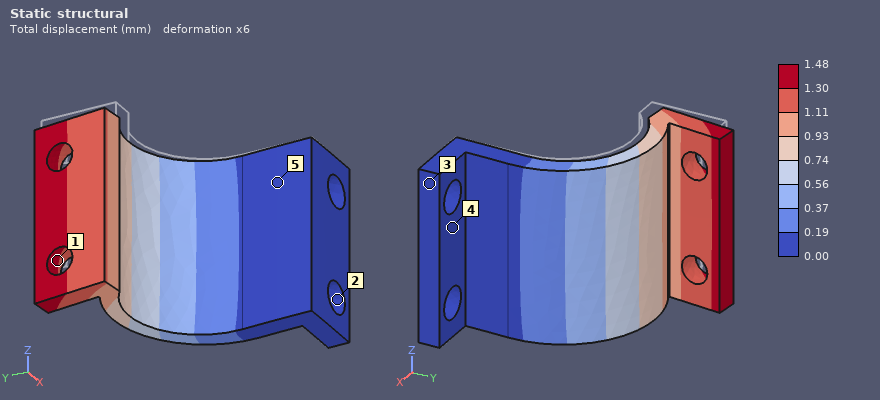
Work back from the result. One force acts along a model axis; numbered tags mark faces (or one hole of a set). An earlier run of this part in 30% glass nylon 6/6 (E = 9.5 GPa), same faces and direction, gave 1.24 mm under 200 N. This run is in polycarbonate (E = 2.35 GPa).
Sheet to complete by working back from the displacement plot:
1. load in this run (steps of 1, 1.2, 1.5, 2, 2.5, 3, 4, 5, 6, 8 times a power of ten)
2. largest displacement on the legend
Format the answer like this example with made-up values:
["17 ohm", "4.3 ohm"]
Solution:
["60 N", "1.48 mm"]
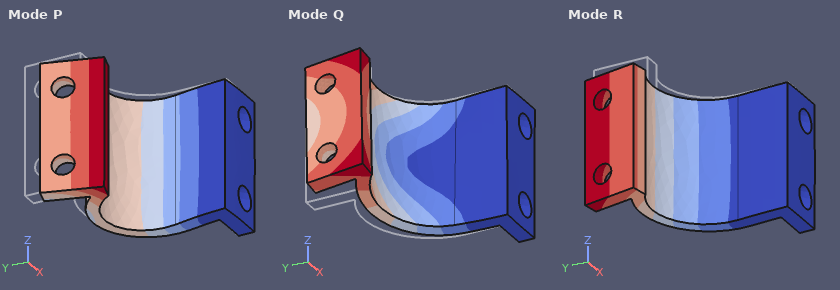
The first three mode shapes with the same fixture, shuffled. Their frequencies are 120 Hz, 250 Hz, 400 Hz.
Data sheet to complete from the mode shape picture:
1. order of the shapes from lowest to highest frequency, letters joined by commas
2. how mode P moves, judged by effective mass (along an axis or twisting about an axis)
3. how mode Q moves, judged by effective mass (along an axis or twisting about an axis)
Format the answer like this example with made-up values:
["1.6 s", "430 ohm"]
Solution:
["R, Q, P", "along X", "along Z"]
